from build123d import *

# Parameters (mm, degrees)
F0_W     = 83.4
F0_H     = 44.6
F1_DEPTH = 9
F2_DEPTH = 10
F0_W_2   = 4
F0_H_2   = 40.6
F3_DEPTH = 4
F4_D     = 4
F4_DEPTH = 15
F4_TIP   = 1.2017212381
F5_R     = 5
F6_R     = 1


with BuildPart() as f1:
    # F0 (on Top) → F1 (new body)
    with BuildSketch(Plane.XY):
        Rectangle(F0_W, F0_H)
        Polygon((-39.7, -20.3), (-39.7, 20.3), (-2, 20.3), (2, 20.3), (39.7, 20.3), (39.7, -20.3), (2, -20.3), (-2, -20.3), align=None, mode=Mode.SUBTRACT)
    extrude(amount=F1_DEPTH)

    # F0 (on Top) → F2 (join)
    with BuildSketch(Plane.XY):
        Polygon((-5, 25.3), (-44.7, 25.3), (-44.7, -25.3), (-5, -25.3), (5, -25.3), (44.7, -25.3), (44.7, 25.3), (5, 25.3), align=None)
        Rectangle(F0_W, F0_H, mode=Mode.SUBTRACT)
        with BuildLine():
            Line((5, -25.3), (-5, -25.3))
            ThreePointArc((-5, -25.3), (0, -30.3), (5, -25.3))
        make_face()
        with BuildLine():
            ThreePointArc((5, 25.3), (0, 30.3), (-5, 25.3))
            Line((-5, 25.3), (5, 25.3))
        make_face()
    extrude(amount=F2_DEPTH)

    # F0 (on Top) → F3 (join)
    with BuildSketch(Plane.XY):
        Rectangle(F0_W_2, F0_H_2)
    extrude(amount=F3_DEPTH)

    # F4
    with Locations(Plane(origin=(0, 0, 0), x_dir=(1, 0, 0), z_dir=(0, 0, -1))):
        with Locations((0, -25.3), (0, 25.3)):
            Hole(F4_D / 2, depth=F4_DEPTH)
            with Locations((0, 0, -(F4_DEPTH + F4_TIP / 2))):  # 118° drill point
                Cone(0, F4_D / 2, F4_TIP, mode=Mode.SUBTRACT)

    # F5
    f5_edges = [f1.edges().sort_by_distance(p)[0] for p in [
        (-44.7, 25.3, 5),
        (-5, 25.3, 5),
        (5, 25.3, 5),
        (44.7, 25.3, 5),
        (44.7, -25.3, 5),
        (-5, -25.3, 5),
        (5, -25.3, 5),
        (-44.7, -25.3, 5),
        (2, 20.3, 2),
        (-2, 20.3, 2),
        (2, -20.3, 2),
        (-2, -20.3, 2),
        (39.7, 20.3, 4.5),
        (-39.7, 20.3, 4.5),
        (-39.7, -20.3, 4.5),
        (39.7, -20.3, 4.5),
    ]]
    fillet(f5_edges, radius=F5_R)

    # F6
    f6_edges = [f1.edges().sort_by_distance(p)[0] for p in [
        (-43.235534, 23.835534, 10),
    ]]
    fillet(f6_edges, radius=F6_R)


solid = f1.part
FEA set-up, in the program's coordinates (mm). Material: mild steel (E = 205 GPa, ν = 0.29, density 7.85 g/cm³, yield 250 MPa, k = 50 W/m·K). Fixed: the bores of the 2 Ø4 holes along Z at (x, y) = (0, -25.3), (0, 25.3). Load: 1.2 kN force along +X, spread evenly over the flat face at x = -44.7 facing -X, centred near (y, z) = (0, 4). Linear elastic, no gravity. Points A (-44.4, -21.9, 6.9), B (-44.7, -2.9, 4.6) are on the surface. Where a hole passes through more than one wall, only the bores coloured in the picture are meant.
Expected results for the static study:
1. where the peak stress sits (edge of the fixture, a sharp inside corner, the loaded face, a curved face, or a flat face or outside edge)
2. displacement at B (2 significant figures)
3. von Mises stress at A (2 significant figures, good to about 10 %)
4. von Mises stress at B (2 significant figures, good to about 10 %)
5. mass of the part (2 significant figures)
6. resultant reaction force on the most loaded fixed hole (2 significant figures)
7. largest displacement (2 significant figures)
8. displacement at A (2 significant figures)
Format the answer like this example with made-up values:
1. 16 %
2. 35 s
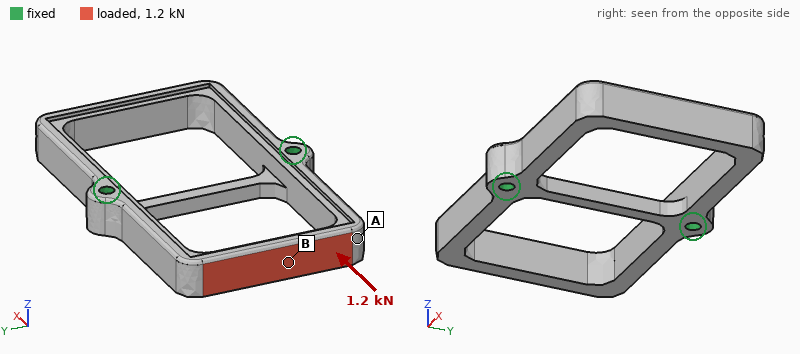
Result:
1. a curved face
2. 30 µm
3. 15 MPa
4. 82 MPa
5. 110 g
6. 620 N
7. 31 µm
8. 4.9 µm
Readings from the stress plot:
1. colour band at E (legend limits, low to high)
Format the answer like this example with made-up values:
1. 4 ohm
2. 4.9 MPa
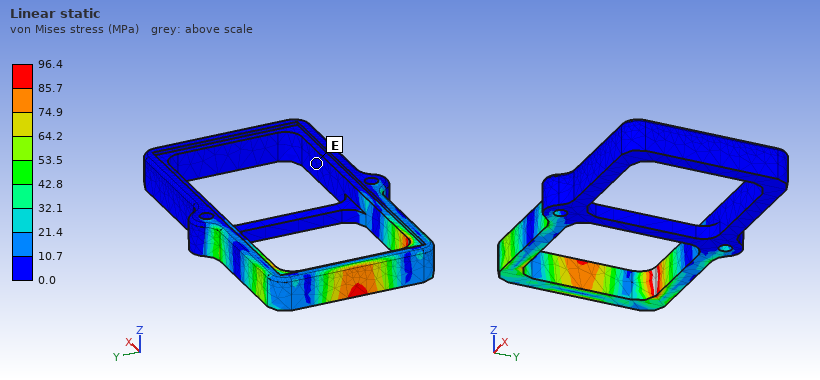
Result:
1. 0.0 to 10.7 MPa
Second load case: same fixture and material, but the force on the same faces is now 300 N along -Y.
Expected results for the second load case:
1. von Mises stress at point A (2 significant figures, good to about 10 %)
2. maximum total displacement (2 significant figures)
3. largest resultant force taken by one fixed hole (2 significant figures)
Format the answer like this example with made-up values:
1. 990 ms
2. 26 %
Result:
1. 14 MPa
2. 43 µm
3. 210 N
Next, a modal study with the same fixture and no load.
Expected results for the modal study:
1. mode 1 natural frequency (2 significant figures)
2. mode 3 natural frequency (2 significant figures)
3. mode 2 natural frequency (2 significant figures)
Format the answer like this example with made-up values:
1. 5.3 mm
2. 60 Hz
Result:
1. 2500 Hz
2. 2600 Hz
3. 2600 Hz
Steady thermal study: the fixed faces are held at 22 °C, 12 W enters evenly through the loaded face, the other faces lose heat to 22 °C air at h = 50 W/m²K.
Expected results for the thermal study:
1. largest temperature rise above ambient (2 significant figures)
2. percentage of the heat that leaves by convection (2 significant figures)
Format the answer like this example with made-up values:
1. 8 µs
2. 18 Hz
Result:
1. 75 K
2. 51 %
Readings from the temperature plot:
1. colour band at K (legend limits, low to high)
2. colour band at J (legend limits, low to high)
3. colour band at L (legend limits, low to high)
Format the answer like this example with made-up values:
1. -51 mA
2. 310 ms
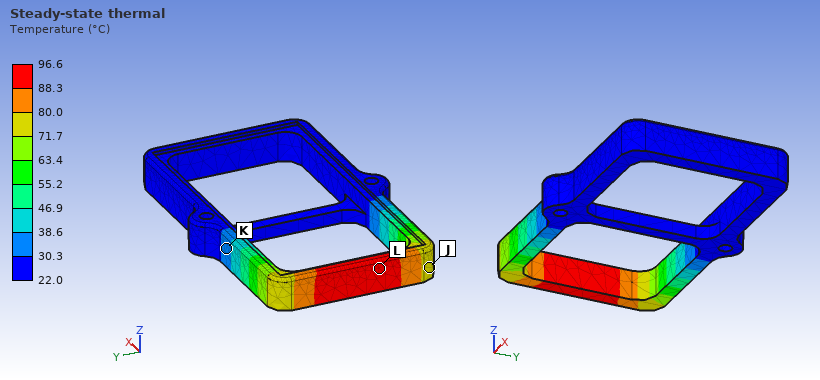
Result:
1. 30.3 to 38.6 °C
2. 71.7 to 80.0 °C
3. 88.3 to 96.6 °C
